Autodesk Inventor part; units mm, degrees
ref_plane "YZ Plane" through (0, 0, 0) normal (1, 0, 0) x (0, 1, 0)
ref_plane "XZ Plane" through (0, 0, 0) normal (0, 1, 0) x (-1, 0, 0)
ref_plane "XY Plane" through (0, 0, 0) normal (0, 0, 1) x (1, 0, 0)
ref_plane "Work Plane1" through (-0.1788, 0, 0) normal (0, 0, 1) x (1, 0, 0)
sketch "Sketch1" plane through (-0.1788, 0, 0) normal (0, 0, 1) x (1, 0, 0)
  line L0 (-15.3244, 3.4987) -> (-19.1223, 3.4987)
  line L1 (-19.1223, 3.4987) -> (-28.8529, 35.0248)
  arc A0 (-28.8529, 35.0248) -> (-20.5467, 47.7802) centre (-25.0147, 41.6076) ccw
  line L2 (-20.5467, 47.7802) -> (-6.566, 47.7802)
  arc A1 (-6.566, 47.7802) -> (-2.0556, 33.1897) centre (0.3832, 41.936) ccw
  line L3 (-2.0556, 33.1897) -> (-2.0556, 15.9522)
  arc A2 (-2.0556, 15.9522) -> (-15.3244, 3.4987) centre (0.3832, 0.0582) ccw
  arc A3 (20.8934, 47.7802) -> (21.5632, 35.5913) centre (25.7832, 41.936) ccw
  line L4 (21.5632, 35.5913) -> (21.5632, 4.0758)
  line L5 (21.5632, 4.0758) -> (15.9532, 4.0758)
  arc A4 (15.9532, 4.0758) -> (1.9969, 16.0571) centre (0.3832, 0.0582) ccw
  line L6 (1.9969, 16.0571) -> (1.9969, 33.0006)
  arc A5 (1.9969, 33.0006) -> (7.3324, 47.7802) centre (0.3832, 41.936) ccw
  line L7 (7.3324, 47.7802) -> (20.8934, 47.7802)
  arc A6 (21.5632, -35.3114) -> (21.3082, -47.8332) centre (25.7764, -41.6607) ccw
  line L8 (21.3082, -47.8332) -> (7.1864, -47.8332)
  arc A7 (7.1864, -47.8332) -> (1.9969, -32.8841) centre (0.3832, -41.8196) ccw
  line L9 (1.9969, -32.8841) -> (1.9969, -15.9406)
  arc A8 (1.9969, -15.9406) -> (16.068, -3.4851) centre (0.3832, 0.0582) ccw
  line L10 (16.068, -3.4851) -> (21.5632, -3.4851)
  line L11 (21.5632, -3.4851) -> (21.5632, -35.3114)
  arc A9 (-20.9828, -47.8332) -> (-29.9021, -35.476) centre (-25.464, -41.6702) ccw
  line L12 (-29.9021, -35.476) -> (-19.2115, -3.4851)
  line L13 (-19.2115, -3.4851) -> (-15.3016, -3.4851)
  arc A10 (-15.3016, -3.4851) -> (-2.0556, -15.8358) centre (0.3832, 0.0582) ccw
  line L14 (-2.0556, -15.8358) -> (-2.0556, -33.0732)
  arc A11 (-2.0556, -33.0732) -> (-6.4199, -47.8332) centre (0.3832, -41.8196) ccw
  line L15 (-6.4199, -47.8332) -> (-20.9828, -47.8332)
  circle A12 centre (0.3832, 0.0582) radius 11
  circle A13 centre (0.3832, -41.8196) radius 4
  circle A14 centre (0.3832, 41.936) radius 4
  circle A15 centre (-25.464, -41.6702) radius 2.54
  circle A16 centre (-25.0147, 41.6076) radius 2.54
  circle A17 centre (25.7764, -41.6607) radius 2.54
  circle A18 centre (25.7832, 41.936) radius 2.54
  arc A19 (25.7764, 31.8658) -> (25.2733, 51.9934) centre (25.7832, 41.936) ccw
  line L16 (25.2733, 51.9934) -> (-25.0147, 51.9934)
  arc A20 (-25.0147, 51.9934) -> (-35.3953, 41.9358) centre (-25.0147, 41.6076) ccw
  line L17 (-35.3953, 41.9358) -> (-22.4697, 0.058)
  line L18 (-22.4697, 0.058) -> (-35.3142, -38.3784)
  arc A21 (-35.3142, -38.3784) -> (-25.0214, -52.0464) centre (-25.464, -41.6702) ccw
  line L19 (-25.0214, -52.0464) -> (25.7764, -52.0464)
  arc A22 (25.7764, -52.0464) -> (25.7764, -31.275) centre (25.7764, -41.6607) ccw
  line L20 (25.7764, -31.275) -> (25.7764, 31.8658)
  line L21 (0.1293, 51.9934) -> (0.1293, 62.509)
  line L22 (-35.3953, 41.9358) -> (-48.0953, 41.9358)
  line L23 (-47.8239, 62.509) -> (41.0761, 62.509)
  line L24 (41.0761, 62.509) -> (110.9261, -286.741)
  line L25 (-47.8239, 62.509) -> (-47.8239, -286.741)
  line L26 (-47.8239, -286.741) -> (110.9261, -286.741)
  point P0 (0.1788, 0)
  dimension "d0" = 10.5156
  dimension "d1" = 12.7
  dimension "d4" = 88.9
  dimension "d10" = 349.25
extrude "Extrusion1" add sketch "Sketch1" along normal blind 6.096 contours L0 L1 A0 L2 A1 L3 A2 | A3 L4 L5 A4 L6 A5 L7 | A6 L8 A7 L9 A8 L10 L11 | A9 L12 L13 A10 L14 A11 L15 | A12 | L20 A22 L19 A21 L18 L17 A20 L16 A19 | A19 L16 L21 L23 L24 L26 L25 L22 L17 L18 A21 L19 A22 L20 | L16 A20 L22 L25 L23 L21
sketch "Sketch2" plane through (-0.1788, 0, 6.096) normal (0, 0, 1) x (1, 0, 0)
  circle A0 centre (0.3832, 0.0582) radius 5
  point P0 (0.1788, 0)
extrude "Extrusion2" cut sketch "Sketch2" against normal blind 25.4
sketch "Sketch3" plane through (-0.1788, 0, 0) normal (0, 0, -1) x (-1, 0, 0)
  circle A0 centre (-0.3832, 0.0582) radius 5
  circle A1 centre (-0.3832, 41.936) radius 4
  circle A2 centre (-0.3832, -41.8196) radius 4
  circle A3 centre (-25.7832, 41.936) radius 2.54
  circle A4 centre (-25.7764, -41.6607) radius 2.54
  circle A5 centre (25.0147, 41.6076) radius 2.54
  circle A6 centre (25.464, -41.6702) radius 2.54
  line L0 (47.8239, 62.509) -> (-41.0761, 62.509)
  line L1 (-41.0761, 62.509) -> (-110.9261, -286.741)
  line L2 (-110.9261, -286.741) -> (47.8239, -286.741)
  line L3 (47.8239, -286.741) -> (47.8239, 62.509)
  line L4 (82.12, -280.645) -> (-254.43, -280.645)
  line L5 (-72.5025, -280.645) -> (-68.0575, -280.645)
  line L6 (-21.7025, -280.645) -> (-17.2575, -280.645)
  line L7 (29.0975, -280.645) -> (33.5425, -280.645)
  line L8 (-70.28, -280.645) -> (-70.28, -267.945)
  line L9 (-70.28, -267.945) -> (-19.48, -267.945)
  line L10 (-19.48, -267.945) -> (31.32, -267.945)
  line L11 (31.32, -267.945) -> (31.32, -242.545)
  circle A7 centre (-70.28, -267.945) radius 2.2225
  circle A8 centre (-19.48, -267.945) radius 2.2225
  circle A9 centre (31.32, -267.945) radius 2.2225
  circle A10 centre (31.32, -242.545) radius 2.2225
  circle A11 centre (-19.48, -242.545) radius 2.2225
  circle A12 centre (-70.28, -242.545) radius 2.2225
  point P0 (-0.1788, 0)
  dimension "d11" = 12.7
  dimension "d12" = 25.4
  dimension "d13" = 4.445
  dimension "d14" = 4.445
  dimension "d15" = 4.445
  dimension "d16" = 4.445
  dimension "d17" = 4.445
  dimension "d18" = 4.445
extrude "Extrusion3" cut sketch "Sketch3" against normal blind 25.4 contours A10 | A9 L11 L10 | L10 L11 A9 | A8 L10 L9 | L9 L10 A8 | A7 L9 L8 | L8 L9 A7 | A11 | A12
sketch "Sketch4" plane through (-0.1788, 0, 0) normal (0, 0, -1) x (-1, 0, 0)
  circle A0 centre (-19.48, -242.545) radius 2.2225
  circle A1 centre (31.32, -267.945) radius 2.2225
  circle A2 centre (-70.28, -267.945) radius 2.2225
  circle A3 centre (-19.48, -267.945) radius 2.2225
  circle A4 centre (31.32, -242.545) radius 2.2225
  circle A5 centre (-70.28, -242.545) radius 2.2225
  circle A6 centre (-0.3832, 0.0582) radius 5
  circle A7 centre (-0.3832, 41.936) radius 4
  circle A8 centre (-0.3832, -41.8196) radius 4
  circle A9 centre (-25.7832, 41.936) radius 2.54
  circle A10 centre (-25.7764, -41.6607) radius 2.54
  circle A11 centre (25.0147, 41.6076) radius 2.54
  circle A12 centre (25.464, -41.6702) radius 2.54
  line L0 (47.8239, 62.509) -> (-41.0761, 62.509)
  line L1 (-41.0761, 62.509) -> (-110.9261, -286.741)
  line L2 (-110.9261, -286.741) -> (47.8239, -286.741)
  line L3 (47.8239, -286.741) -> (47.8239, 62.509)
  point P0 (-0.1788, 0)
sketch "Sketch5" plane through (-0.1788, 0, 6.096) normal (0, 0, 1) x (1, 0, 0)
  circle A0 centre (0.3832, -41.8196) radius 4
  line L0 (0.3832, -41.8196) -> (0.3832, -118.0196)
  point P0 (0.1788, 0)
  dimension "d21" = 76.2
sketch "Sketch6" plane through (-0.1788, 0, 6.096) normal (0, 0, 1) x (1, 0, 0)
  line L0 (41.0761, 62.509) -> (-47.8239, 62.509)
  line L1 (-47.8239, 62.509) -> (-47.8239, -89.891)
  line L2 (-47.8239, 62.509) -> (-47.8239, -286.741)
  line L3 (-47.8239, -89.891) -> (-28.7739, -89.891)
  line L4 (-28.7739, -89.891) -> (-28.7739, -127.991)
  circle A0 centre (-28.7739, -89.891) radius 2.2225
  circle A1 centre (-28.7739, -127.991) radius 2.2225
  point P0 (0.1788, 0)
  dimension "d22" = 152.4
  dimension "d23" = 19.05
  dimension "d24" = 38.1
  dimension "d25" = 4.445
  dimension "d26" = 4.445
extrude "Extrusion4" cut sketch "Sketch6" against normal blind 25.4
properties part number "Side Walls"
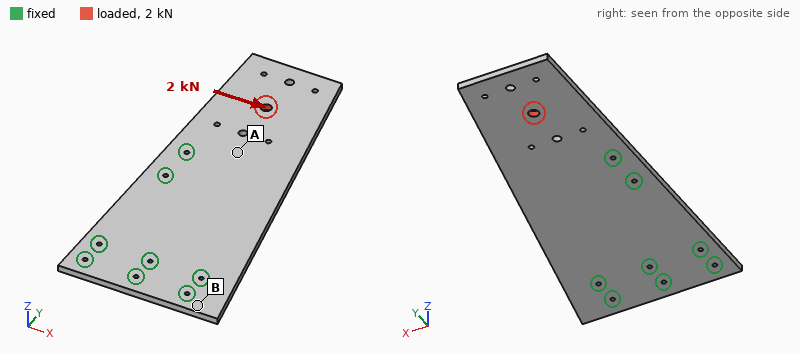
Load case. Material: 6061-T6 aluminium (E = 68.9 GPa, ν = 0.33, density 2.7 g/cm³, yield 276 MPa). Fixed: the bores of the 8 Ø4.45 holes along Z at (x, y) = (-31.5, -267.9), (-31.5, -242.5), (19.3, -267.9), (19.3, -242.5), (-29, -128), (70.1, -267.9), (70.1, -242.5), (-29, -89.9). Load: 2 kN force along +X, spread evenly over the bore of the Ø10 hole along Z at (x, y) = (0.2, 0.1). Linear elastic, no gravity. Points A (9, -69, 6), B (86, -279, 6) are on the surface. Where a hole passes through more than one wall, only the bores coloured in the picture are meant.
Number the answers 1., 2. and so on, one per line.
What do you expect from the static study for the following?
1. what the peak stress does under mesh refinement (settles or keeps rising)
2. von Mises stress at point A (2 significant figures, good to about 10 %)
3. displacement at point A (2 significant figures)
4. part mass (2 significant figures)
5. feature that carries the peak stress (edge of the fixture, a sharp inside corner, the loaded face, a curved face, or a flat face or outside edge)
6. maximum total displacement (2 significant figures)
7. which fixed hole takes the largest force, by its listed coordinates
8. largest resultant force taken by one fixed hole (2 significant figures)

1. keeps rising
2. 6.6 MPa
3. 11 µm
4. 710 g
5. edge of the fixture
6. 59 µm
7. (-29, -89.9)
8. 2.7 kN
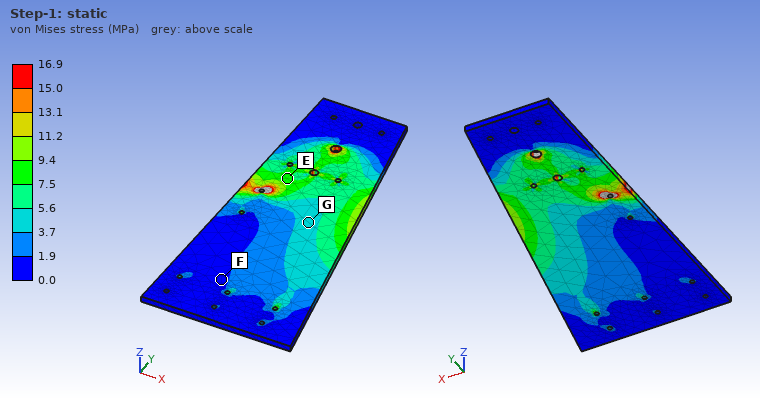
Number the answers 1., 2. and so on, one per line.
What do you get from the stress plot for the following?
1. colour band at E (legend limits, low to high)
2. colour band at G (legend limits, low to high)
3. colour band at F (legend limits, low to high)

1. 7.5 to 9.4 MPa
2. 3.7 to 5.6 MPa
3. 0.0 to 1.9 MPa
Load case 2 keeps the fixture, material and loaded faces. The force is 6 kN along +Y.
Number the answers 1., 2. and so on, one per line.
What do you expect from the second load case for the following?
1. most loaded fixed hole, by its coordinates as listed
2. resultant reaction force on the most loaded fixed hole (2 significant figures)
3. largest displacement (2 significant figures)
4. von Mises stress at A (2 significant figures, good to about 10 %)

1. (-29, -89.9)
2. 2.8 kN
3. 27 µm
4. 8.2 MPa
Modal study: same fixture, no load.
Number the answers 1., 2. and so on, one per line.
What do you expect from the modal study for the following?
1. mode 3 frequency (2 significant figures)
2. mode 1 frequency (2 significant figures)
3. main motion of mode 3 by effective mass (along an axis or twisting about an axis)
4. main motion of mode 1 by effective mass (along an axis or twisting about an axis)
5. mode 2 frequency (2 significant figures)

1. 870 Hz
2. 200 Hz
3. along Z
4. along Z
5. 470 Hz
